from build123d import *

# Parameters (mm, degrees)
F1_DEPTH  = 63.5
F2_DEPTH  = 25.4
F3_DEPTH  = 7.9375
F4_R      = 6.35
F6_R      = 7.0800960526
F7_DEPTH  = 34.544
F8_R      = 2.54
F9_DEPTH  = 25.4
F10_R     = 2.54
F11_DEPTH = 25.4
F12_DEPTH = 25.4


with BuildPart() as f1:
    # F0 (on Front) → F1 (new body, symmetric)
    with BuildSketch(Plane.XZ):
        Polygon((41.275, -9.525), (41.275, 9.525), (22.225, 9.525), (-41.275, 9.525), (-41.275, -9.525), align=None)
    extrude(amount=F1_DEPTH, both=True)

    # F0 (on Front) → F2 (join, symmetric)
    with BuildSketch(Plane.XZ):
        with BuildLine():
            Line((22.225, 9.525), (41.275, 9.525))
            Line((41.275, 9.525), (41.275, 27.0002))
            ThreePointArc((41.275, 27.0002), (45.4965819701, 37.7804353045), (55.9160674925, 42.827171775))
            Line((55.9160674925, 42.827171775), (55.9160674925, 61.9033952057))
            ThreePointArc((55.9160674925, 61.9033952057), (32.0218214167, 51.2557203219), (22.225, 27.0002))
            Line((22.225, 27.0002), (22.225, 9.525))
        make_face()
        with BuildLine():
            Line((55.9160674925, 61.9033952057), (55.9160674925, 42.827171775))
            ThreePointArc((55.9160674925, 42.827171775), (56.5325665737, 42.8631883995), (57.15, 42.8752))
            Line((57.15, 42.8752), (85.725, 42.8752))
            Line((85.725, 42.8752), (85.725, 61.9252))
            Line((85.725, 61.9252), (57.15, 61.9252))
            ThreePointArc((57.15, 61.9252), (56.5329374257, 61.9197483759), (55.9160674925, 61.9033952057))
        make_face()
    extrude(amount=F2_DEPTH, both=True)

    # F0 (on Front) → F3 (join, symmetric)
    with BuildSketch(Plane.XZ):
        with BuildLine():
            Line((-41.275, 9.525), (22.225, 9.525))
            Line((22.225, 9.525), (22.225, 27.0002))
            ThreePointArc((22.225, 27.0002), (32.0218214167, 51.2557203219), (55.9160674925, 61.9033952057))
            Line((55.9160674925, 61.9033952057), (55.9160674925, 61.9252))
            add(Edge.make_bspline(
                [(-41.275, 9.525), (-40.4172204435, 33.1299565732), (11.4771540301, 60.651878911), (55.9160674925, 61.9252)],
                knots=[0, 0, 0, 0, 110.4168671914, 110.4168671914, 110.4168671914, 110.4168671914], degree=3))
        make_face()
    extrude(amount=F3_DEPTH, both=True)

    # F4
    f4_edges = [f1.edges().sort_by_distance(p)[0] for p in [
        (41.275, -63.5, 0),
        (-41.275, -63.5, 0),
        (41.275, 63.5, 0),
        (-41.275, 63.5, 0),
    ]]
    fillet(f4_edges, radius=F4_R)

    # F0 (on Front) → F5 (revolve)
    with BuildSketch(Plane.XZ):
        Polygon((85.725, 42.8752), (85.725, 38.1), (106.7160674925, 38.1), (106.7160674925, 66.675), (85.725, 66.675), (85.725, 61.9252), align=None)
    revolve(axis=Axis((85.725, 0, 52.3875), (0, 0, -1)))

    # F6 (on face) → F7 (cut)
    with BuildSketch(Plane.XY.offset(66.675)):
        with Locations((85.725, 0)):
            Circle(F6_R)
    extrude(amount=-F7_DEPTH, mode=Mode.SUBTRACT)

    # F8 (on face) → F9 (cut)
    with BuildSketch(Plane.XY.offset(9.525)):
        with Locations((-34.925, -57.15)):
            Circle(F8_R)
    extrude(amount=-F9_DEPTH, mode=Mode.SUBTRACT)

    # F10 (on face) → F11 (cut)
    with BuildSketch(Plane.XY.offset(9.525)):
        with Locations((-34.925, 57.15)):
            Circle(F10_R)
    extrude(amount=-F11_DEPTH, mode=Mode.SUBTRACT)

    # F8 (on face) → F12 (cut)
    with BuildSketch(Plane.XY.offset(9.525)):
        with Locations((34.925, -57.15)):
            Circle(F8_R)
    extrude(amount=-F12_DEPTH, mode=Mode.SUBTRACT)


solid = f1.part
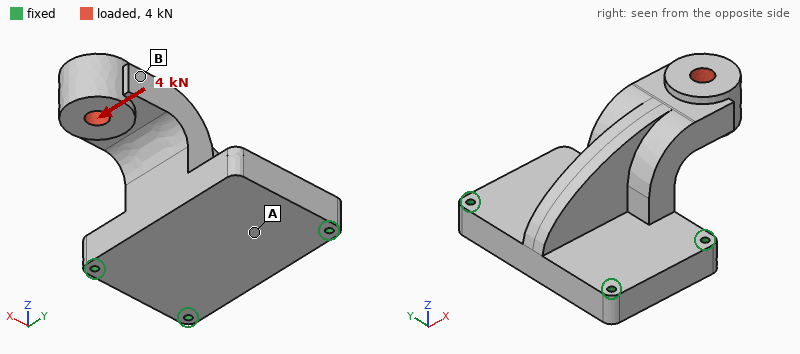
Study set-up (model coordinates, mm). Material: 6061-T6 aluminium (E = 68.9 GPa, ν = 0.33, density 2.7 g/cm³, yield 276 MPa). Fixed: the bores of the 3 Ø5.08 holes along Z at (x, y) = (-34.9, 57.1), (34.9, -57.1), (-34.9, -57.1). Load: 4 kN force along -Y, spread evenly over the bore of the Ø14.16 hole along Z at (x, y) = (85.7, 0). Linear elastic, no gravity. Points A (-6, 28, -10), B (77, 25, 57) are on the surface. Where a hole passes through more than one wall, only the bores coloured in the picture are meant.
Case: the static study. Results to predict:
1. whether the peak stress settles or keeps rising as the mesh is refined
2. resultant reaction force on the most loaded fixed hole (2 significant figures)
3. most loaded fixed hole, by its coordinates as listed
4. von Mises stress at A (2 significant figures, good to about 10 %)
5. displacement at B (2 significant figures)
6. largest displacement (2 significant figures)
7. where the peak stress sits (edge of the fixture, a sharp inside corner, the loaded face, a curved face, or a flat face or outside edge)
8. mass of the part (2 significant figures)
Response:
keeps rising
3.4 kN
(-34.9, 57.1)
12 MPa
0.19 mm
0.27 mm
edge of the fixture
910 g
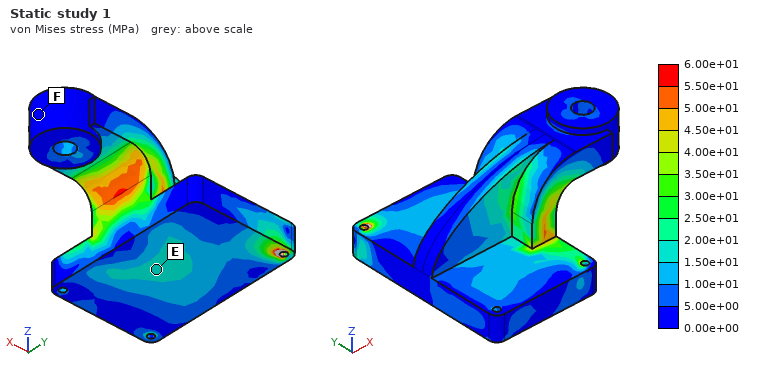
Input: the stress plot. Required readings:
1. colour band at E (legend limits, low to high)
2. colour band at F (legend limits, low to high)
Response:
1.50e+01 to 2.00e+01 MPa
0.00e+00 to 5.00e+00 MPa
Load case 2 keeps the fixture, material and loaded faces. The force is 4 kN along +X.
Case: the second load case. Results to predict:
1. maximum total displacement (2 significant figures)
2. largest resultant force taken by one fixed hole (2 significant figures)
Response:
0.18 mm
3.0 kN
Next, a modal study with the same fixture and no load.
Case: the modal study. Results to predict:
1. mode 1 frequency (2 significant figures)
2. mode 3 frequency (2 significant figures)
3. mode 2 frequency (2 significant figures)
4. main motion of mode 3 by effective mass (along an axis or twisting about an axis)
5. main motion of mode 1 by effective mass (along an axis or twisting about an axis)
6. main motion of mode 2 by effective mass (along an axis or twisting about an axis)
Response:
1200 Hz
3200 Hz
2000 Hz
along Z
along Z
along Y
